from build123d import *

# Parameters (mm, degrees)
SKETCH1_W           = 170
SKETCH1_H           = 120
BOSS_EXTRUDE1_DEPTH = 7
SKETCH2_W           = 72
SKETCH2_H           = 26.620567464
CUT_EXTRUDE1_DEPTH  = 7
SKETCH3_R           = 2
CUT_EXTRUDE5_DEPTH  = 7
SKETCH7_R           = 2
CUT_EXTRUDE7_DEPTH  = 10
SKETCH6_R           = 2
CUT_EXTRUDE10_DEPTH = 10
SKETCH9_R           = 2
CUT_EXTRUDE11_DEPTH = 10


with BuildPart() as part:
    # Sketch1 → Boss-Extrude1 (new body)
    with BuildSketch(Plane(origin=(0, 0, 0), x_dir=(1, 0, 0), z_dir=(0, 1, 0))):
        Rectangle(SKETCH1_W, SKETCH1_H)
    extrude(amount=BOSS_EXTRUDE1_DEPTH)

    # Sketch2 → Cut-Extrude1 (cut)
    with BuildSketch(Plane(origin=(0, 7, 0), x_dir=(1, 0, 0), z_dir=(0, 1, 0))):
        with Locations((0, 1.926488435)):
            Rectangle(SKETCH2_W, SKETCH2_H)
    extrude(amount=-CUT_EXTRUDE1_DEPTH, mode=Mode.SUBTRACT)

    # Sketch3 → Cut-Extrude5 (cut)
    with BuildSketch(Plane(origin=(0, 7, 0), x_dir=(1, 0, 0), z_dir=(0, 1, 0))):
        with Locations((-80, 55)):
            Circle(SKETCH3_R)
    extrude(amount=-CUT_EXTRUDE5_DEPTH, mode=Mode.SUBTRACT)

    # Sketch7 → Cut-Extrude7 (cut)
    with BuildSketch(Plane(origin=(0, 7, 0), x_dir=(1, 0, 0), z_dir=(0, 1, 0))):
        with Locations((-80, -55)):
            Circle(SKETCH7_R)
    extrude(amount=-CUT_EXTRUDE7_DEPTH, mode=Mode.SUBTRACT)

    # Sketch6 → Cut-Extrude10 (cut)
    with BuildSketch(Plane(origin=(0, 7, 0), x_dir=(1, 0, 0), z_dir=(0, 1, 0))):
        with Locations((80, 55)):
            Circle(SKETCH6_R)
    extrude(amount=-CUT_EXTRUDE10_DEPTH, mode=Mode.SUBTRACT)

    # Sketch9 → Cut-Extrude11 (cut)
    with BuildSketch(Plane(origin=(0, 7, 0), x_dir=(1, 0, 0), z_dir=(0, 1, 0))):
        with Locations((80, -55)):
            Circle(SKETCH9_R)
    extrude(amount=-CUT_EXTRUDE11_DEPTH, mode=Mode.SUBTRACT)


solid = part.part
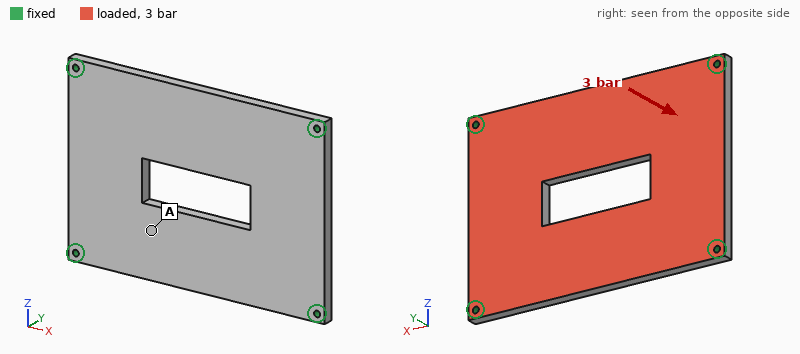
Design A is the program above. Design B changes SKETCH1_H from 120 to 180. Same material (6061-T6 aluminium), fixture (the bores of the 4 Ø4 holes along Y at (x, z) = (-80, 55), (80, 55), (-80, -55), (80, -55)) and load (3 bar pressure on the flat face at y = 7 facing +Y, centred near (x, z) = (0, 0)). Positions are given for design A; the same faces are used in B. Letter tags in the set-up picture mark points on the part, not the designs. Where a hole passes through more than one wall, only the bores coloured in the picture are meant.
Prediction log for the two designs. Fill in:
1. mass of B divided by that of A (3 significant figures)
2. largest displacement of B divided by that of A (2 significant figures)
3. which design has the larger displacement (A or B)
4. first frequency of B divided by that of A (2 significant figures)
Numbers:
1.55
0.90
A
1.0
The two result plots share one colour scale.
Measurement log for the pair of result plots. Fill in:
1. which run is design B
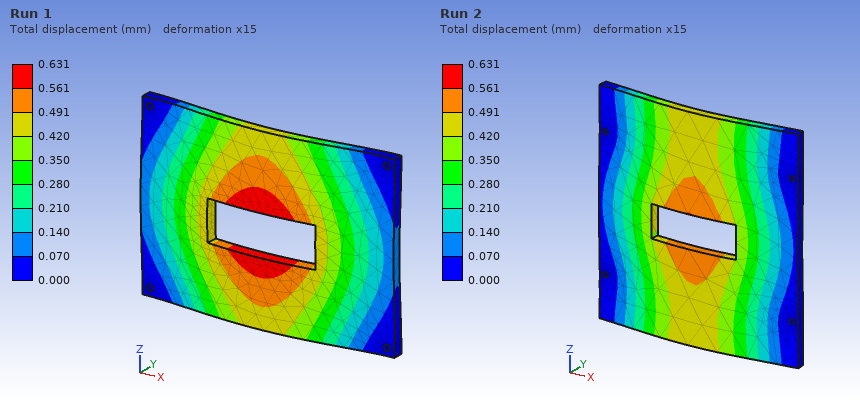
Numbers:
Run 2
